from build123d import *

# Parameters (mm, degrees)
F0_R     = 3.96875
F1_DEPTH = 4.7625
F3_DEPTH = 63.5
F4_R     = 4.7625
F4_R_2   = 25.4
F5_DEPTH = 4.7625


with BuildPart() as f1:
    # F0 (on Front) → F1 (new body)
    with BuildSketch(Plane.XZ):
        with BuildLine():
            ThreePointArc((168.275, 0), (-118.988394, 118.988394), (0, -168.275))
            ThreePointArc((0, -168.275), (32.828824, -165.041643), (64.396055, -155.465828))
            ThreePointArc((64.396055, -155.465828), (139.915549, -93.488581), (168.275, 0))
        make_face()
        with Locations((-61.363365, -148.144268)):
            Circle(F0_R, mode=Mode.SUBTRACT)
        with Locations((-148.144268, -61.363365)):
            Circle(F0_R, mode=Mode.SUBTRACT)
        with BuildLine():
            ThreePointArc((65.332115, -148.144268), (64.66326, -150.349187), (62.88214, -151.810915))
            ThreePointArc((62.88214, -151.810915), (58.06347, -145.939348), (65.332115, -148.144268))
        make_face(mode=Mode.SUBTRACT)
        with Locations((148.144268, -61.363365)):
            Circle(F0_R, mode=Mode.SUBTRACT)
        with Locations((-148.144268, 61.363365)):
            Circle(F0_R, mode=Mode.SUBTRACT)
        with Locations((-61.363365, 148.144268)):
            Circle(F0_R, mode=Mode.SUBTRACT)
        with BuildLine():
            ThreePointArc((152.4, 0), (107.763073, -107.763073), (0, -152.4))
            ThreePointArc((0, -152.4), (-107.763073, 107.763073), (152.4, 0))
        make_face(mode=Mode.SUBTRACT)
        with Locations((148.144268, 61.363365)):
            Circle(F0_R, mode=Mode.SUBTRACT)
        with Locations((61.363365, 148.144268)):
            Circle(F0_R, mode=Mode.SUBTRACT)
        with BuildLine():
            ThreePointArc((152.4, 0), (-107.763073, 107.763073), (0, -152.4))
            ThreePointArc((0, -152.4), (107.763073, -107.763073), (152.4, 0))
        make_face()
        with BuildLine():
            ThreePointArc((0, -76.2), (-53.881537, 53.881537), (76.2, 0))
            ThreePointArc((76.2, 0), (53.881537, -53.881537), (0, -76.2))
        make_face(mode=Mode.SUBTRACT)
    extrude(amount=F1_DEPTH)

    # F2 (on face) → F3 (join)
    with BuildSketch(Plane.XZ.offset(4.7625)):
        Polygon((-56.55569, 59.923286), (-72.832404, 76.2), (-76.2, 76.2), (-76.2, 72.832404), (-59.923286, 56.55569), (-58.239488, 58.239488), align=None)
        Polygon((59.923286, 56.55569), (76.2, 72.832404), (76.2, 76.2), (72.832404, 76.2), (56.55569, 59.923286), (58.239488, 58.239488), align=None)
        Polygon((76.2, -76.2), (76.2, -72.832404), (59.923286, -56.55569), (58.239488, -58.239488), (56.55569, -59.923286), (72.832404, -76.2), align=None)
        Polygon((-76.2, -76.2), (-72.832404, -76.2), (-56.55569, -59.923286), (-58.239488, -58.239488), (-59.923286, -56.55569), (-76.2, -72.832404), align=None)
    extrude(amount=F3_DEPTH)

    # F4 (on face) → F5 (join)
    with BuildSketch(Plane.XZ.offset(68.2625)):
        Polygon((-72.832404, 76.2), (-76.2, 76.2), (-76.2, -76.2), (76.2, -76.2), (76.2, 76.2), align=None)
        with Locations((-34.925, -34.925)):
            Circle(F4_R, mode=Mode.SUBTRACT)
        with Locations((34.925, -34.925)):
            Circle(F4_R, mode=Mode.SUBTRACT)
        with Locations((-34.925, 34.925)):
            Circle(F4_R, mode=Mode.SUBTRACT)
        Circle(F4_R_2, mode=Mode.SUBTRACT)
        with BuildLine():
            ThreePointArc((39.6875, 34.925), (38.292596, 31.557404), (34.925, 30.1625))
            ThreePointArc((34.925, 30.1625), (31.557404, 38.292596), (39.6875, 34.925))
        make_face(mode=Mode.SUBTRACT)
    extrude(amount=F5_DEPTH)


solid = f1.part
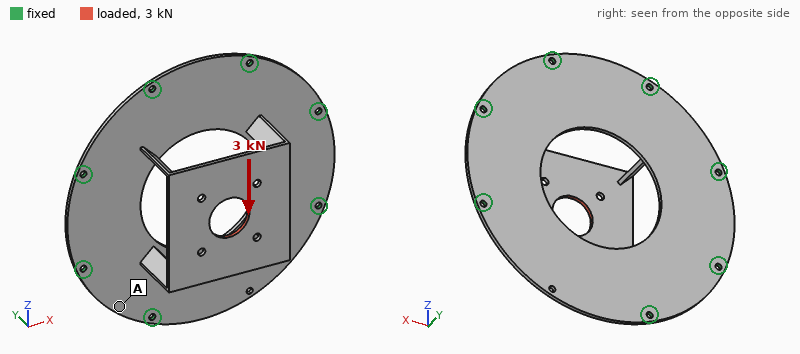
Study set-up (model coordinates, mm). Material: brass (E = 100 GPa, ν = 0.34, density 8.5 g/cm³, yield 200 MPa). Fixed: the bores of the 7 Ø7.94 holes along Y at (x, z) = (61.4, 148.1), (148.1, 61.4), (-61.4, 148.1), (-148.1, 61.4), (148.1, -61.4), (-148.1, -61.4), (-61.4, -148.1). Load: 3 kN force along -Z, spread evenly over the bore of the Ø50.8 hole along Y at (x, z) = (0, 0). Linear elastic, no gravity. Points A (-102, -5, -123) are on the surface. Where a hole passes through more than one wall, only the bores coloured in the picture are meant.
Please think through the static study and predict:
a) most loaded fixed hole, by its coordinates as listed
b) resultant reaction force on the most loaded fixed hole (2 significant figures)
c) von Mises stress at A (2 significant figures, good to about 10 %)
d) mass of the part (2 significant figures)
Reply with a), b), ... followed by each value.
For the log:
a) (-61.4, -148.1)
b) 730 N
c) 13 MPa
d) 3.9 kg
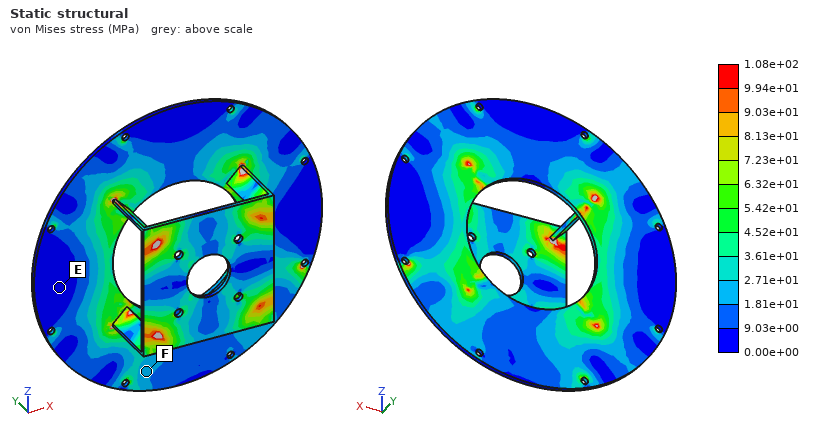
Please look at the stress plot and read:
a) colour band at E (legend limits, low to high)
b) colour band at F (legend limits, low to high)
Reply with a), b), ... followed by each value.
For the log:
a) 0.00e+00 to 9.03e+00 MPa
b) 1.81e+01 to 2.71e+01 MPa
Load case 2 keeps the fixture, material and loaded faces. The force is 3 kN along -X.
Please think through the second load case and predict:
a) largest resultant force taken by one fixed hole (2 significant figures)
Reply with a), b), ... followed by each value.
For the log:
a) 660 N
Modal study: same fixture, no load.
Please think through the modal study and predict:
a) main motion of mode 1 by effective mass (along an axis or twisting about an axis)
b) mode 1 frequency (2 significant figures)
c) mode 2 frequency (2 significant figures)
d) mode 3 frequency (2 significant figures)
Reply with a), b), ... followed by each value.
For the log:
a) along Y
b) 260 Hz
c) 320 Hz
d) 330 Hz
